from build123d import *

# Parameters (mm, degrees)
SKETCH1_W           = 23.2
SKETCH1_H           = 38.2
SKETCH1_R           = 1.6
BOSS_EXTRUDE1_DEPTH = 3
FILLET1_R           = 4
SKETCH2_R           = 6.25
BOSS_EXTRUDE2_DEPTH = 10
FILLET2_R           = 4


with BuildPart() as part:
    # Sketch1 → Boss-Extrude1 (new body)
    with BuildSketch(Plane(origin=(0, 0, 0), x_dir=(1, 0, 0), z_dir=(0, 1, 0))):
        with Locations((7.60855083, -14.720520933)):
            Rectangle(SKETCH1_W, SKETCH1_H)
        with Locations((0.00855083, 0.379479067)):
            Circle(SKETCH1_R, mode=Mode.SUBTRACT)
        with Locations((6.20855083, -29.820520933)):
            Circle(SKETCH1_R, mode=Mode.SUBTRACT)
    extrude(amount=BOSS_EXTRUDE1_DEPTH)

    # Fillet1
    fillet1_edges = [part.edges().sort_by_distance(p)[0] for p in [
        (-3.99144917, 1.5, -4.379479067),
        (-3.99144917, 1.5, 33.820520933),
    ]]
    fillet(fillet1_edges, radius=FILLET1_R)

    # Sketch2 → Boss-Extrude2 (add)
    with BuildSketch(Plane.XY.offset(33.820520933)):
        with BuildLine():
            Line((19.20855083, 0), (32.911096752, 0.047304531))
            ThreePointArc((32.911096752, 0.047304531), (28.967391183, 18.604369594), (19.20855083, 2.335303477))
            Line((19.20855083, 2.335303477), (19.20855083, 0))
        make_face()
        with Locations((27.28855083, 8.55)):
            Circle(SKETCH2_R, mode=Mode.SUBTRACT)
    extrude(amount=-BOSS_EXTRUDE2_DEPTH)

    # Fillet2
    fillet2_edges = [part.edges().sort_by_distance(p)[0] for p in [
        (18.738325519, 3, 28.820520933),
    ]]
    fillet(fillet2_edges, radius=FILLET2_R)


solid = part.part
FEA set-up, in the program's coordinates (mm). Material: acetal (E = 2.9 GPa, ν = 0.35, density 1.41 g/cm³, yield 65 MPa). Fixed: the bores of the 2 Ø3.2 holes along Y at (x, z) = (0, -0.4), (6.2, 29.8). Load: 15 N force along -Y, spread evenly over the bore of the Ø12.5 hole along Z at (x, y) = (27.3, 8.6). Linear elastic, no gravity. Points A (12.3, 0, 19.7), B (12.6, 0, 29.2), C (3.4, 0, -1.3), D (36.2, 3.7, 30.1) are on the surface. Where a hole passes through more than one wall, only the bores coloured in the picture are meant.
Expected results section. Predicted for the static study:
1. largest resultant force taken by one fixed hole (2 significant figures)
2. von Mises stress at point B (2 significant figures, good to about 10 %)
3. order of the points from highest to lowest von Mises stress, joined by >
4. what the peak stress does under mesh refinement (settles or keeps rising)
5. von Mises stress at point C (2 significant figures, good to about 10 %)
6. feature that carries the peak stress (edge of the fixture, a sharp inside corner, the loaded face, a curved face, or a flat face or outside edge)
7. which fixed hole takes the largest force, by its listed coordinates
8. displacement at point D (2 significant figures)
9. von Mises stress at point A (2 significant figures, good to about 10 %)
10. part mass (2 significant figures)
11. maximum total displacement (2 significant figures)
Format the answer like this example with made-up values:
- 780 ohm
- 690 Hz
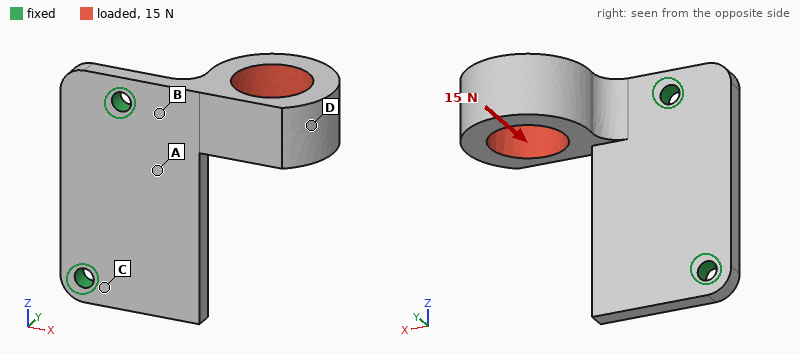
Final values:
- 16 N
- 8.5 MPa
- B > A > C > D
- keeps rising
- 2.4 MPa
- edge of the fixture
- (6.2, 29.8)
- 0.57 mm
- 4.7 MPa
- 6.5 g
- 0.63 mm
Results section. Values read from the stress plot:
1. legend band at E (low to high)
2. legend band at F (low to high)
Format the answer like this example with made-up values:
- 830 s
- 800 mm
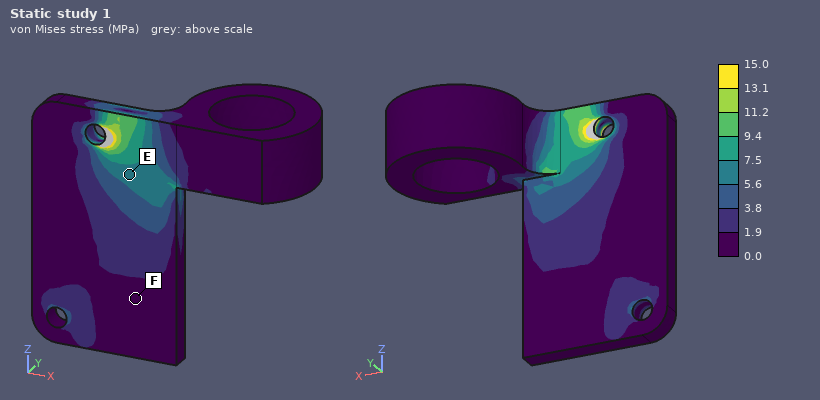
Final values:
- 5.6 to 7.5 MPa
- 0.0 to 1.9 MPa
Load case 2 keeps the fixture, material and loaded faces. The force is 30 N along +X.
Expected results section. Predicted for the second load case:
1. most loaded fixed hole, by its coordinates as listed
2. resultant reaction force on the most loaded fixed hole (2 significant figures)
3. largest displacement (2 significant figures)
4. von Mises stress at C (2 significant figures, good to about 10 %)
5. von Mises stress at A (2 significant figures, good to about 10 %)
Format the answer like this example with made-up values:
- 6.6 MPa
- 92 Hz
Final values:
- (6.2, 29.8)
- 29 N
- 0.56 mm
- 1.8 MPa
- 4.0 MPa
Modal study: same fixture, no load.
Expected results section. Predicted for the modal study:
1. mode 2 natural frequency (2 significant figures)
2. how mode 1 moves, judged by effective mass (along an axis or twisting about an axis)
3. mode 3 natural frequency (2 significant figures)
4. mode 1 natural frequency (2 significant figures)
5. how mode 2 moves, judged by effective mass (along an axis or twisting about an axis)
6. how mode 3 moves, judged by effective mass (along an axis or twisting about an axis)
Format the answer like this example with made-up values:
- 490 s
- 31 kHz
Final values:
- 1200 Hz
- along Y
- 2300 Hz
- 500 Hz
- along Z
- along Y
